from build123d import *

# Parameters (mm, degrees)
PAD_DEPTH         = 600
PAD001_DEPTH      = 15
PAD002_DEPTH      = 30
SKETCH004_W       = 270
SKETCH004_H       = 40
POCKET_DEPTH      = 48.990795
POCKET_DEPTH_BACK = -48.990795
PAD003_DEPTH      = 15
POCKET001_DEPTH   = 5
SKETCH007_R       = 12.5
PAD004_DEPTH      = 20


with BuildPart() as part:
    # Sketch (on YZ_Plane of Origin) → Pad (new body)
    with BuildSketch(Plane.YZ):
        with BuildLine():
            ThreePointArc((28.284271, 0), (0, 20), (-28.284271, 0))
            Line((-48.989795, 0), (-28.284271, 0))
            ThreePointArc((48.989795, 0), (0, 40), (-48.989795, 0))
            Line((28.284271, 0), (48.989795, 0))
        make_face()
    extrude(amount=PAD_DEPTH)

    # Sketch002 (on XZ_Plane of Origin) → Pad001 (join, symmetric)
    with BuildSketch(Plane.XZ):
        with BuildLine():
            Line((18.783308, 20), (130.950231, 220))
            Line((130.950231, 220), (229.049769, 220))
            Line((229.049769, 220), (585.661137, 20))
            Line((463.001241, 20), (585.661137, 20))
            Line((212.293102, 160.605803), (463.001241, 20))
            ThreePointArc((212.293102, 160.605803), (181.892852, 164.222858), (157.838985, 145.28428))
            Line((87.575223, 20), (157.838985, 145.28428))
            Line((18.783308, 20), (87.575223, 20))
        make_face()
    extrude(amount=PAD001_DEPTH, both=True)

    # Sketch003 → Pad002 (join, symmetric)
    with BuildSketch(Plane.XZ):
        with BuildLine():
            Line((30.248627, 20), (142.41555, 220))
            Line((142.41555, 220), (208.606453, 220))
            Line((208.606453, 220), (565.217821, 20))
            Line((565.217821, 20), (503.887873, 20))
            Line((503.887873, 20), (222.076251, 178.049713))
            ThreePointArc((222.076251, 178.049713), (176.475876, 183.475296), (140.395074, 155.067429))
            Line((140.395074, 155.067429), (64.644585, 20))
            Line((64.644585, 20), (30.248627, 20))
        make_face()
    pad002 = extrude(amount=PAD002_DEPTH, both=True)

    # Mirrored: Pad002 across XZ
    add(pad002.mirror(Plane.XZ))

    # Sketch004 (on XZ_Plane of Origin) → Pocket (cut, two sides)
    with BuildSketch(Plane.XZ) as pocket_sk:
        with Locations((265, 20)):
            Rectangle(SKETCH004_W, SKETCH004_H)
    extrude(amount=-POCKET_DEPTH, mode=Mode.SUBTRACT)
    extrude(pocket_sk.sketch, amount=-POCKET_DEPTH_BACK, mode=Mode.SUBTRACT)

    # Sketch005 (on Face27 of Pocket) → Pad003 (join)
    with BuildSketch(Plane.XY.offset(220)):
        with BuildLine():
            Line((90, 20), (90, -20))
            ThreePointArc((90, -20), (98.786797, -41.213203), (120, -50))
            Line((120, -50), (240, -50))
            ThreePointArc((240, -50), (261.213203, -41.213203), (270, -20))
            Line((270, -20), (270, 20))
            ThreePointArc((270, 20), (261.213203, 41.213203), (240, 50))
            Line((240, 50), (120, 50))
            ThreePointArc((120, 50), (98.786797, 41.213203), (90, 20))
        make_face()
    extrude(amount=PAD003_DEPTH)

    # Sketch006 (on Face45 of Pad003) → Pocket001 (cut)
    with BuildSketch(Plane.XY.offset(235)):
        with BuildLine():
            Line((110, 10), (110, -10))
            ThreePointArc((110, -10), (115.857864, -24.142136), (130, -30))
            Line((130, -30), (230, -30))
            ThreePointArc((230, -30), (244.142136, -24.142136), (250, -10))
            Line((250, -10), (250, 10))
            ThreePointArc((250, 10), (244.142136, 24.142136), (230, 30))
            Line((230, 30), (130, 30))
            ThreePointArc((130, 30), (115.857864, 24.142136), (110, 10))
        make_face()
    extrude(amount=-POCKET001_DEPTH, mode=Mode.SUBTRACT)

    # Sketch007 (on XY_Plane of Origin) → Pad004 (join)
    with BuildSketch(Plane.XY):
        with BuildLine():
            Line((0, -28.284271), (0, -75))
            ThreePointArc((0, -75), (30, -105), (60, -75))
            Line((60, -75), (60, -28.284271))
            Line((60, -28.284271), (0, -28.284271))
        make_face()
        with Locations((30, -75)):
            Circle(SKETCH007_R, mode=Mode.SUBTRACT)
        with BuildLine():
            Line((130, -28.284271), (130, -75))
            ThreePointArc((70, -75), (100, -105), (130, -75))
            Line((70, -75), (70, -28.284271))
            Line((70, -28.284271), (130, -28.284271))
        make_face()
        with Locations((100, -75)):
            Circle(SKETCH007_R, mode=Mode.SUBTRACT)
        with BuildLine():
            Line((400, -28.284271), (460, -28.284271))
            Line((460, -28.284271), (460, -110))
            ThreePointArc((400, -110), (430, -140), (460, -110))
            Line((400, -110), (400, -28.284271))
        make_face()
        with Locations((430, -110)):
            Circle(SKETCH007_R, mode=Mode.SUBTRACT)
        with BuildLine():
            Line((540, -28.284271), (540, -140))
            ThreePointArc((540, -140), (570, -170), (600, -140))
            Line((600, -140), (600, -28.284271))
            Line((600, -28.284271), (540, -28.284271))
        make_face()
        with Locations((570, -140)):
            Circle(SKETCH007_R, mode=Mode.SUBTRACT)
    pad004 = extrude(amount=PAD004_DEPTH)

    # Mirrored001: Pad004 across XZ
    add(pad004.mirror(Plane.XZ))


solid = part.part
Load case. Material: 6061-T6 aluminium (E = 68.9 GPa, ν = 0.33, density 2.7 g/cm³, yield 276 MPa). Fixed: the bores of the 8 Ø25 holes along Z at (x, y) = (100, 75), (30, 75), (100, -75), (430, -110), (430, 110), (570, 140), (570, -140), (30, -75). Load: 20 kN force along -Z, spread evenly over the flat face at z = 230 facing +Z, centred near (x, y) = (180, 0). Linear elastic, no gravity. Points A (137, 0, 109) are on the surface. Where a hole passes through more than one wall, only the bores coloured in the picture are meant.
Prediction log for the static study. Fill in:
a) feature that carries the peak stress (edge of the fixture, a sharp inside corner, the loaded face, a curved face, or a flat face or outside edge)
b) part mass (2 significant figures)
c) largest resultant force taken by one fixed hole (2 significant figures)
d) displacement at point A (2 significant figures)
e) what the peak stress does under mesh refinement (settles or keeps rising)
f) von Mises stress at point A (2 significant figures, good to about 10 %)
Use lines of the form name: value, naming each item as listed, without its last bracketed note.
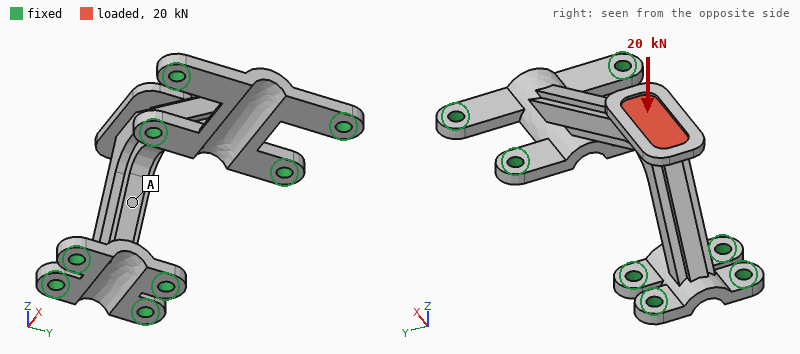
feature that carries the peak stress: edge of the fixture
part mass: 8.4 kg
largest resultant force taken by one fixed hole: 7.0 kN
displacement at point A: 0.038 mm
what the peak stress does under mesh refinement: keeps rising
von Mises stress at point A: 10 MPa
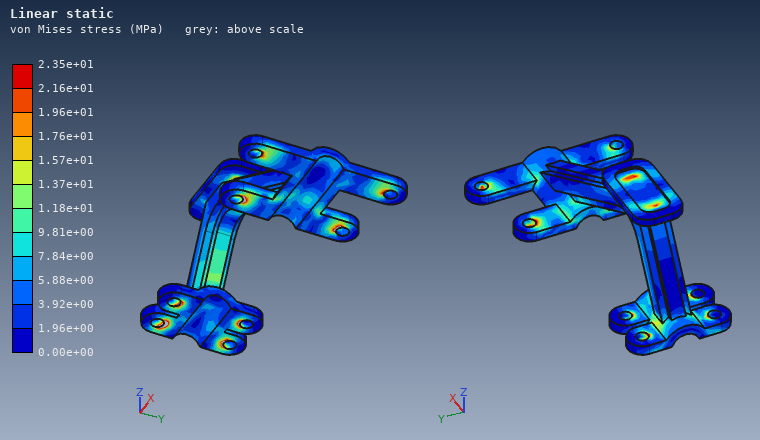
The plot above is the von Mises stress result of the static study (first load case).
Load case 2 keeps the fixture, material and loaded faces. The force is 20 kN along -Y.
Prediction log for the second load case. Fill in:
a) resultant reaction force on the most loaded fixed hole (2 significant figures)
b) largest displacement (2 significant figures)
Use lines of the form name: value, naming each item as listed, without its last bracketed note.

resultant reaction force on the most loaded fixed hole: 17 kN
largest displacement: 1.9 mm
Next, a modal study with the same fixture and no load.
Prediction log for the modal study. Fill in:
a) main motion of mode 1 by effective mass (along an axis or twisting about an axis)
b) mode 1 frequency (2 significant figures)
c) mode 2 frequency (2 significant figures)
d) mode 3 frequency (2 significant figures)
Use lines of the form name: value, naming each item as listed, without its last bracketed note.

main motion of mode 1 by effective mass: along Y
mode 1 frequency: 420 Hz
mode 2 frequency: 980 Hz
mode 3 frequency: 1200 Hz
